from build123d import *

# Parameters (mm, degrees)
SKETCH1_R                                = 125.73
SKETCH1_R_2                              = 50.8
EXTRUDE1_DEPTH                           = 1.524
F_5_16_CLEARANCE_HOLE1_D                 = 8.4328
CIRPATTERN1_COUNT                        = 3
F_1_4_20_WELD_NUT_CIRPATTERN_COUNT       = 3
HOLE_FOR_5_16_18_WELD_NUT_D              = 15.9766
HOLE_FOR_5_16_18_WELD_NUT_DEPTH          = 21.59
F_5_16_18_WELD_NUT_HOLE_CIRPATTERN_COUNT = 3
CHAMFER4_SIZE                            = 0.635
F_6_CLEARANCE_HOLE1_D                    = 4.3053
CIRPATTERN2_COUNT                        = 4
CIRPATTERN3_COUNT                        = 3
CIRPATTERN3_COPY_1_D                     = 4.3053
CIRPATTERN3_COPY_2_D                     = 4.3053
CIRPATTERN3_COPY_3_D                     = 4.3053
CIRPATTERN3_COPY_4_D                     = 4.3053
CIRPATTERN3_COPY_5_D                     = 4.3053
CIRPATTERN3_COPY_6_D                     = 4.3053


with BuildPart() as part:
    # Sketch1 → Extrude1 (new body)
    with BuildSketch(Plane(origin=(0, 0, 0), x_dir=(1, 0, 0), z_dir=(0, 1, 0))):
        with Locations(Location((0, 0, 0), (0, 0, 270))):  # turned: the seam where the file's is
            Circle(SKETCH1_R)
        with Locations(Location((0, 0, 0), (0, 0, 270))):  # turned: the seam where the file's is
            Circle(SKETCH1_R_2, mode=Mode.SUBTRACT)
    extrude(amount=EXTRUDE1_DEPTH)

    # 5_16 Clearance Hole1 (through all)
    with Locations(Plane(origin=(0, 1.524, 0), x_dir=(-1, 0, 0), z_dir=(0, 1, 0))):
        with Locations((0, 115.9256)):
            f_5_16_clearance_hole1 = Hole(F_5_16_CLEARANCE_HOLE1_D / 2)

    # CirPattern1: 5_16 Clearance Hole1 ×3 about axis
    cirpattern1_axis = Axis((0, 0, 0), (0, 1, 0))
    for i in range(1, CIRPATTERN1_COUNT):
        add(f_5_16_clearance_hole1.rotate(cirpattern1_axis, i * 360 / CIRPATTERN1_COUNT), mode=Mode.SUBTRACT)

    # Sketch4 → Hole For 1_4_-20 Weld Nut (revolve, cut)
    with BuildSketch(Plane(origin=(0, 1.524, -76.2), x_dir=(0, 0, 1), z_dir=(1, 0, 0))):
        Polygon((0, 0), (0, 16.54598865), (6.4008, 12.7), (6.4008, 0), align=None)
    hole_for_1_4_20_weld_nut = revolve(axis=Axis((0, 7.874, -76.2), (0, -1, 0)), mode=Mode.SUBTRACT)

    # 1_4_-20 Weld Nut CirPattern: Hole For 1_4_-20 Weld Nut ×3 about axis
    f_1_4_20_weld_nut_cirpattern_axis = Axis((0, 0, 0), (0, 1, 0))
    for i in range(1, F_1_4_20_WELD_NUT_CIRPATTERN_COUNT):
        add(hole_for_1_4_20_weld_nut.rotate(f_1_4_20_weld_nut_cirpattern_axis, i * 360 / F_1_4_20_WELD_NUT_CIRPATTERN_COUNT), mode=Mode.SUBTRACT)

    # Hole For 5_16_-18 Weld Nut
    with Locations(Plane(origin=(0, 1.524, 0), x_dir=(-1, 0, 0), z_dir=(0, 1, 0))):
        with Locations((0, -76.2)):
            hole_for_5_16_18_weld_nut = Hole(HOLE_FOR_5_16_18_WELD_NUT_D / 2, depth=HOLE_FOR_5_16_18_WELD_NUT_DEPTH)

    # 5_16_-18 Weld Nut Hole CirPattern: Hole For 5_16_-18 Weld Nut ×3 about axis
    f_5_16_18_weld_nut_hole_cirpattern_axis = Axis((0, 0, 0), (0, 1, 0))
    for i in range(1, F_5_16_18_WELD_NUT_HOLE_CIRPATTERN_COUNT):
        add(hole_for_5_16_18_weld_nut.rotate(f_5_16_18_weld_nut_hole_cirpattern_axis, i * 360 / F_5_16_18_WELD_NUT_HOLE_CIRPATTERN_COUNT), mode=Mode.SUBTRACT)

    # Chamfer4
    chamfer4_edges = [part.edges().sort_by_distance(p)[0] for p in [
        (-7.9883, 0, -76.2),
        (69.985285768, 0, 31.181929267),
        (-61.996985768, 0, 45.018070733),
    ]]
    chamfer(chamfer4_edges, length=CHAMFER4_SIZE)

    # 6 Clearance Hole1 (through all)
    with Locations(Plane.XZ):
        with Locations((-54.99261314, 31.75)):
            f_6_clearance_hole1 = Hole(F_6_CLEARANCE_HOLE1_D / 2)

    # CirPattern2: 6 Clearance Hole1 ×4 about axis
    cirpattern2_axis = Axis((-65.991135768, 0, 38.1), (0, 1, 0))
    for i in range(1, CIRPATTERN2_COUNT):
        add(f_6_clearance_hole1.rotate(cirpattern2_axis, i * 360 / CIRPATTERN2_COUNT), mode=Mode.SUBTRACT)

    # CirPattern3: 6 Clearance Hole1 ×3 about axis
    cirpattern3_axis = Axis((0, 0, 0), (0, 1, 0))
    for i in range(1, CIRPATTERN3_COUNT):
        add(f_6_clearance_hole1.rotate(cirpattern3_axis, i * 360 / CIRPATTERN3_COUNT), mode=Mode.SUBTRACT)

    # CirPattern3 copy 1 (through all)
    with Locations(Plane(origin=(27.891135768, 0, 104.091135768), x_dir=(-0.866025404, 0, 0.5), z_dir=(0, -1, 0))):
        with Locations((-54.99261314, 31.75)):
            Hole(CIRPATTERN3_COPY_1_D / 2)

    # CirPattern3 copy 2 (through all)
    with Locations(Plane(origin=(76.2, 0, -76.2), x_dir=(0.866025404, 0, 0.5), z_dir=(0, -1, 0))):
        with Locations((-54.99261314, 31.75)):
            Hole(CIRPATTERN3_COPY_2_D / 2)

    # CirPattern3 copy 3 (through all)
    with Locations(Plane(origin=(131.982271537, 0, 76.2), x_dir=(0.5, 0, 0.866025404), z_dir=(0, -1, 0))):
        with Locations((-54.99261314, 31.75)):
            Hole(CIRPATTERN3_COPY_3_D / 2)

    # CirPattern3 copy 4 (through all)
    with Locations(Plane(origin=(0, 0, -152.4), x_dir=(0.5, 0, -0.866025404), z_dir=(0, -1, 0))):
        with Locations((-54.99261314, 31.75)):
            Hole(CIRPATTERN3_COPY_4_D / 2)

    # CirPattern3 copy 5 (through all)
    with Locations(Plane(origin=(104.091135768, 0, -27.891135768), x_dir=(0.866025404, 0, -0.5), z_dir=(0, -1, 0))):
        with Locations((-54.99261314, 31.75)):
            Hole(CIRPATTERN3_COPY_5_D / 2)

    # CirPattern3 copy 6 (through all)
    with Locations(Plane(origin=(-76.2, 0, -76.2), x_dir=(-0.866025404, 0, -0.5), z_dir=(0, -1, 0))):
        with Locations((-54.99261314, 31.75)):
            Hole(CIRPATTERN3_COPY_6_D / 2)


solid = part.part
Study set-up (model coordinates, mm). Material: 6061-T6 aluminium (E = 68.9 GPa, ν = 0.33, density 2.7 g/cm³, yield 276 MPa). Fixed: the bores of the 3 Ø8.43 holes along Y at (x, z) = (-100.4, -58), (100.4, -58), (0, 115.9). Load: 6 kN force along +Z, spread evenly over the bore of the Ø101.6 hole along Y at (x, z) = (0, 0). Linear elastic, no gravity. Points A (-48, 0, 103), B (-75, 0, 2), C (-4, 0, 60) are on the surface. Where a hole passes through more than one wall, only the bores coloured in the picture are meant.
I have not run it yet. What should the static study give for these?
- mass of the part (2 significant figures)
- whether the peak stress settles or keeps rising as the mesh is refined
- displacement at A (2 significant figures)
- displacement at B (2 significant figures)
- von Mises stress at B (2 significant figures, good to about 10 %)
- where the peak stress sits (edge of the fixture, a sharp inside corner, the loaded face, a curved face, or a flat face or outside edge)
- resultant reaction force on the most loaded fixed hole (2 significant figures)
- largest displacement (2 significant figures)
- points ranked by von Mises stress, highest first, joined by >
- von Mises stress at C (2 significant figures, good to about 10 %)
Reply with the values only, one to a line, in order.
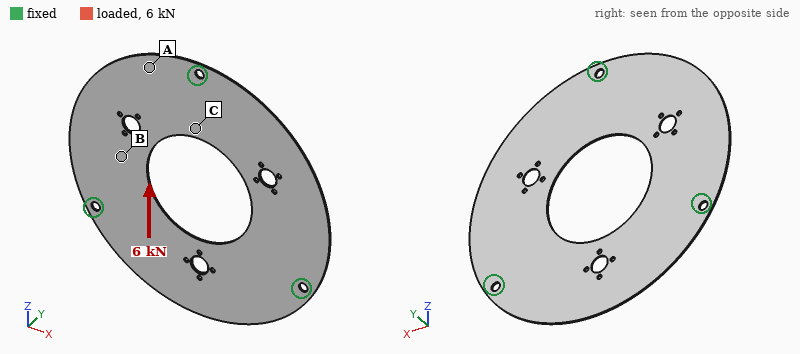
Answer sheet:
170 g
keeps rising
23 µm
34 µm
14 MPa
edge of the fixture
2.1 kN
67 µm
C > B > A
23 MPa
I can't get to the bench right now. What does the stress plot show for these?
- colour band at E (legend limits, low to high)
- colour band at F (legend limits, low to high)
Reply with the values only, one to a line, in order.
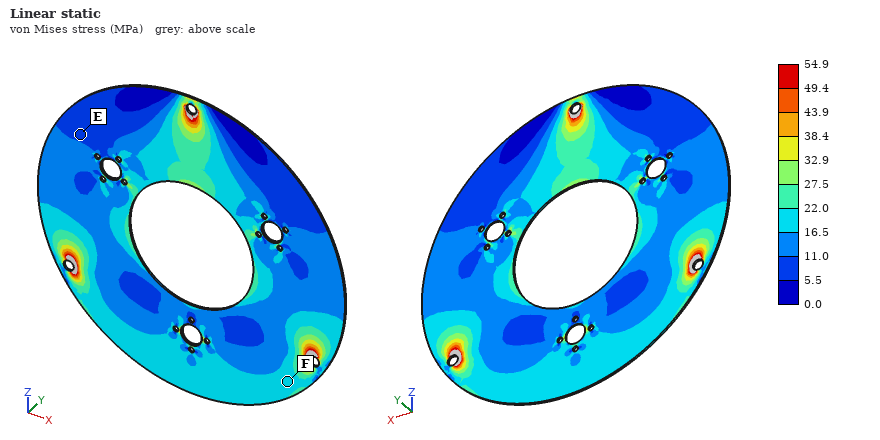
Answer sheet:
5.5 to 11.0 MPa
16.5 to 22.0 MPa
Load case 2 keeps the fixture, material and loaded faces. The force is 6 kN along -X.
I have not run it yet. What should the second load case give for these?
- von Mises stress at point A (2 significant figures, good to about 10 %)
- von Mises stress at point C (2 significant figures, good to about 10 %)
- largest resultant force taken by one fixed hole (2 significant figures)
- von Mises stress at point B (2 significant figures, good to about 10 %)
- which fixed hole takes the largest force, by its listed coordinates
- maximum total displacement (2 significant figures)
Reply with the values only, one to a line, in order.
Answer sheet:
20 MPa
11 MPa
2.3 kN
14 MPa
(0, 115.9)
60 µm
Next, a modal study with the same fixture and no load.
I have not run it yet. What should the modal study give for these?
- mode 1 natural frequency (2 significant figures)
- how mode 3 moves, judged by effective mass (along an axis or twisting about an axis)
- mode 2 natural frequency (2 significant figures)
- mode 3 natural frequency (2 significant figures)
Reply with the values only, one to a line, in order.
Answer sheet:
140 Hz
along Y
140 Hz
170 Hz
